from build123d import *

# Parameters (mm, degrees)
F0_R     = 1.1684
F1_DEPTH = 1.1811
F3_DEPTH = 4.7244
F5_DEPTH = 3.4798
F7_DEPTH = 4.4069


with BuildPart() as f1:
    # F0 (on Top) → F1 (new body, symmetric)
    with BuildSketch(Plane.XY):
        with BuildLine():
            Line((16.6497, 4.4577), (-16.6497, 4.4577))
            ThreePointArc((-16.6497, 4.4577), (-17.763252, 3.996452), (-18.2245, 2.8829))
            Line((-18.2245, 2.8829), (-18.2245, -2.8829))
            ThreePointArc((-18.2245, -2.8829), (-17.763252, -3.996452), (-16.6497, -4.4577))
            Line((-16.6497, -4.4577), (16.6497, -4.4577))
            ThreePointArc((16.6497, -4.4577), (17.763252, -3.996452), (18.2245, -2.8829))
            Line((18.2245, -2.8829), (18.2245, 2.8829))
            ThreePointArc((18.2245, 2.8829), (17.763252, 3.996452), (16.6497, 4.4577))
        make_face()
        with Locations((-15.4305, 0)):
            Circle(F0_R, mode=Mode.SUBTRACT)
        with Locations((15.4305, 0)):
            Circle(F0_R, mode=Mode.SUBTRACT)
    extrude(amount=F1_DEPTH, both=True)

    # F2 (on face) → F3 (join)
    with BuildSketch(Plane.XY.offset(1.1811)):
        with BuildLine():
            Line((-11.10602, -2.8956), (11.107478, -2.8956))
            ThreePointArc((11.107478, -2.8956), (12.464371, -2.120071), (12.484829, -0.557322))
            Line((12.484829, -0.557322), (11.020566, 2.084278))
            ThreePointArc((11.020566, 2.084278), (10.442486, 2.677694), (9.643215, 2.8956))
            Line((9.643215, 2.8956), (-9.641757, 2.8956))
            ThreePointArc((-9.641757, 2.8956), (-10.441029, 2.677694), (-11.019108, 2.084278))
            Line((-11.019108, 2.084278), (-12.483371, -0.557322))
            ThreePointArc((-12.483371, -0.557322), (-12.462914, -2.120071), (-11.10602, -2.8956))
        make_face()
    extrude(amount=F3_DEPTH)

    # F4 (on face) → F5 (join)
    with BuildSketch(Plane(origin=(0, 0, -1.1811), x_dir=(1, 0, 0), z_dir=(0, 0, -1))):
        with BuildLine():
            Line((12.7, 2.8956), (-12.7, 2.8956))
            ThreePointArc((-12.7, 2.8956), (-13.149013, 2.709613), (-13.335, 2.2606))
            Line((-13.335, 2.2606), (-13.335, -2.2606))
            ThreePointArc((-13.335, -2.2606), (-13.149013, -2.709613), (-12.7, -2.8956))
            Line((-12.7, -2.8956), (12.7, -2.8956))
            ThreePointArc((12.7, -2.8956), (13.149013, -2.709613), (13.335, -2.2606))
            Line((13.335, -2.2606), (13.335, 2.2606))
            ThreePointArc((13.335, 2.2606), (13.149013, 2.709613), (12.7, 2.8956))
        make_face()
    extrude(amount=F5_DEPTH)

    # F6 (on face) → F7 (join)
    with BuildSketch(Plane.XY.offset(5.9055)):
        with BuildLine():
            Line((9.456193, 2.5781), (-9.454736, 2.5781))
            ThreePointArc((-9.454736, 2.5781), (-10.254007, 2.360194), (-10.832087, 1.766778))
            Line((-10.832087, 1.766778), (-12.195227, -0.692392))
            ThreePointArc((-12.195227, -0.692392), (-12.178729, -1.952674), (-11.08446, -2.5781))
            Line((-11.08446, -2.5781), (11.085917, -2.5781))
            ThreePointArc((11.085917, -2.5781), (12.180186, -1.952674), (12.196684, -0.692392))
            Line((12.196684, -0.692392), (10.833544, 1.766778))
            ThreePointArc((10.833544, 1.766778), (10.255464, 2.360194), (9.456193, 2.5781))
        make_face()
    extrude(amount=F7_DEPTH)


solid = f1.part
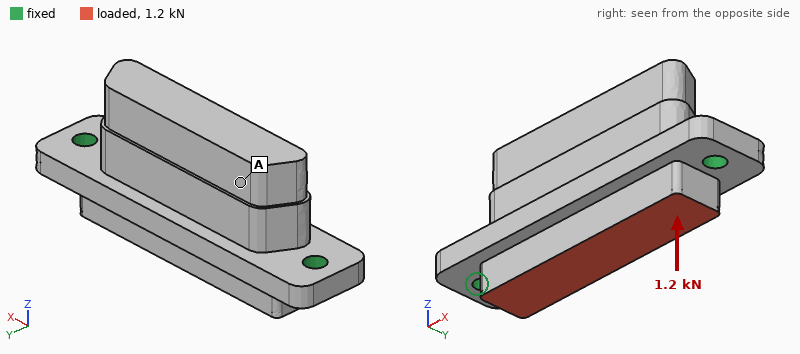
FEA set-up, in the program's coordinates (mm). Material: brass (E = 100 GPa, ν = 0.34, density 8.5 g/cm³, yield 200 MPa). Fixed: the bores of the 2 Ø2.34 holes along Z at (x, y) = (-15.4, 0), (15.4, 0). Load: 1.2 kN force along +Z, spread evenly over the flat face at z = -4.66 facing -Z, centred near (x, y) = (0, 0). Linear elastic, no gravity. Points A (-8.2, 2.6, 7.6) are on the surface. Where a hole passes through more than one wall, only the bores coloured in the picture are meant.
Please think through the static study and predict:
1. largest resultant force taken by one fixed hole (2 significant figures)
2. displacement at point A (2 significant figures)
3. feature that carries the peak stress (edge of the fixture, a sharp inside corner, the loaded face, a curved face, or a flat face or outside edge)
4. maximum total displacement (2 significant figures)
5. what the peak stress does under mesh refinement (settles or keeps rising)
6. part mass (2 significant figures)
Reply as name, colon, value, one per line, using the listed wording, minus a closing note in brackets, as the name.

largest resultant force taken by one fixed hole: 600 N
displacement at point A: 7.8 µm
feature that carries the peak stress: edge of the fixture
maximum total displacement: 9.5 µm
what the peak stress does under mesh refinement: keeps rising
part mass: 21 g
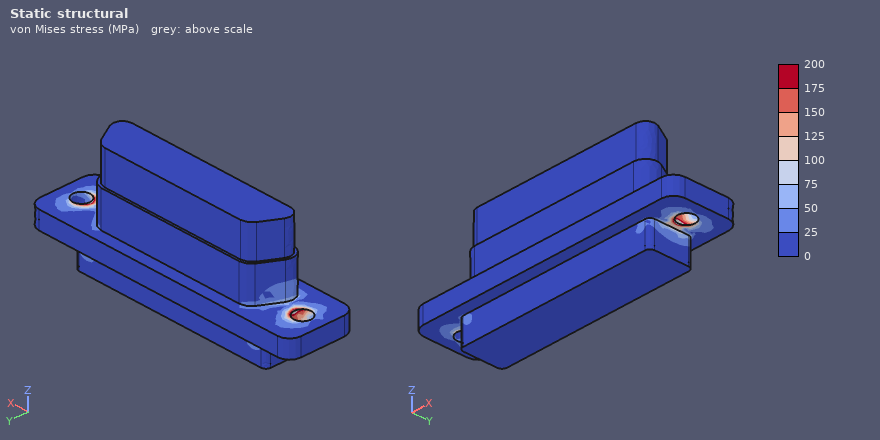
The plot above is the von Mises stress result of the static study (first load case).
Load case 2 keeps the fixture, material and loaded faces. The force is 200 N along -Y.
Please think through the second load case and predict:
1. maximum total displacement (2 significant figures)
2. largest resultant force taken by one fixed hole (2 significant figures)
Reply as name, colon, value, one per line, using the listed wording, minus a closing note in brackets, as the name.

maximum total displacement: 8.2 µm
largest resultant force taken by one fixed hole: 100 N
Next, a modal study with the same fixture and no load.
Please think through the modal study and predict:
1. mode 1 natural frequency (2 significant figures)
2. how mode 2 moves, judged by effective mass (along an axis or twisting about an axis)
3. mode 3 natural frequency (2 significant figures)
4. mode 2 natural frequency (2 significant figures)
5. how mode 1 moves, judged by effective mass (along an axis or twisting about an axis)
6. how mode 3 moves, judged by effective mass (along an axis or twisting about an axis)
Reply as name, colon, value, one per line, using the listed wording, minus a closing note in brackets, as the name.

mode 1 natural frequency: 6400 Hz
how mode 2 moves, judged by effective mass: along Y
mode 3 natural frequency: 14 kHz
mode 2 natural frequency: 13 kHz
how mode 1 moves, judged by effective mass: along Y
how mode 3 moves, judged by effective mass: along Z
